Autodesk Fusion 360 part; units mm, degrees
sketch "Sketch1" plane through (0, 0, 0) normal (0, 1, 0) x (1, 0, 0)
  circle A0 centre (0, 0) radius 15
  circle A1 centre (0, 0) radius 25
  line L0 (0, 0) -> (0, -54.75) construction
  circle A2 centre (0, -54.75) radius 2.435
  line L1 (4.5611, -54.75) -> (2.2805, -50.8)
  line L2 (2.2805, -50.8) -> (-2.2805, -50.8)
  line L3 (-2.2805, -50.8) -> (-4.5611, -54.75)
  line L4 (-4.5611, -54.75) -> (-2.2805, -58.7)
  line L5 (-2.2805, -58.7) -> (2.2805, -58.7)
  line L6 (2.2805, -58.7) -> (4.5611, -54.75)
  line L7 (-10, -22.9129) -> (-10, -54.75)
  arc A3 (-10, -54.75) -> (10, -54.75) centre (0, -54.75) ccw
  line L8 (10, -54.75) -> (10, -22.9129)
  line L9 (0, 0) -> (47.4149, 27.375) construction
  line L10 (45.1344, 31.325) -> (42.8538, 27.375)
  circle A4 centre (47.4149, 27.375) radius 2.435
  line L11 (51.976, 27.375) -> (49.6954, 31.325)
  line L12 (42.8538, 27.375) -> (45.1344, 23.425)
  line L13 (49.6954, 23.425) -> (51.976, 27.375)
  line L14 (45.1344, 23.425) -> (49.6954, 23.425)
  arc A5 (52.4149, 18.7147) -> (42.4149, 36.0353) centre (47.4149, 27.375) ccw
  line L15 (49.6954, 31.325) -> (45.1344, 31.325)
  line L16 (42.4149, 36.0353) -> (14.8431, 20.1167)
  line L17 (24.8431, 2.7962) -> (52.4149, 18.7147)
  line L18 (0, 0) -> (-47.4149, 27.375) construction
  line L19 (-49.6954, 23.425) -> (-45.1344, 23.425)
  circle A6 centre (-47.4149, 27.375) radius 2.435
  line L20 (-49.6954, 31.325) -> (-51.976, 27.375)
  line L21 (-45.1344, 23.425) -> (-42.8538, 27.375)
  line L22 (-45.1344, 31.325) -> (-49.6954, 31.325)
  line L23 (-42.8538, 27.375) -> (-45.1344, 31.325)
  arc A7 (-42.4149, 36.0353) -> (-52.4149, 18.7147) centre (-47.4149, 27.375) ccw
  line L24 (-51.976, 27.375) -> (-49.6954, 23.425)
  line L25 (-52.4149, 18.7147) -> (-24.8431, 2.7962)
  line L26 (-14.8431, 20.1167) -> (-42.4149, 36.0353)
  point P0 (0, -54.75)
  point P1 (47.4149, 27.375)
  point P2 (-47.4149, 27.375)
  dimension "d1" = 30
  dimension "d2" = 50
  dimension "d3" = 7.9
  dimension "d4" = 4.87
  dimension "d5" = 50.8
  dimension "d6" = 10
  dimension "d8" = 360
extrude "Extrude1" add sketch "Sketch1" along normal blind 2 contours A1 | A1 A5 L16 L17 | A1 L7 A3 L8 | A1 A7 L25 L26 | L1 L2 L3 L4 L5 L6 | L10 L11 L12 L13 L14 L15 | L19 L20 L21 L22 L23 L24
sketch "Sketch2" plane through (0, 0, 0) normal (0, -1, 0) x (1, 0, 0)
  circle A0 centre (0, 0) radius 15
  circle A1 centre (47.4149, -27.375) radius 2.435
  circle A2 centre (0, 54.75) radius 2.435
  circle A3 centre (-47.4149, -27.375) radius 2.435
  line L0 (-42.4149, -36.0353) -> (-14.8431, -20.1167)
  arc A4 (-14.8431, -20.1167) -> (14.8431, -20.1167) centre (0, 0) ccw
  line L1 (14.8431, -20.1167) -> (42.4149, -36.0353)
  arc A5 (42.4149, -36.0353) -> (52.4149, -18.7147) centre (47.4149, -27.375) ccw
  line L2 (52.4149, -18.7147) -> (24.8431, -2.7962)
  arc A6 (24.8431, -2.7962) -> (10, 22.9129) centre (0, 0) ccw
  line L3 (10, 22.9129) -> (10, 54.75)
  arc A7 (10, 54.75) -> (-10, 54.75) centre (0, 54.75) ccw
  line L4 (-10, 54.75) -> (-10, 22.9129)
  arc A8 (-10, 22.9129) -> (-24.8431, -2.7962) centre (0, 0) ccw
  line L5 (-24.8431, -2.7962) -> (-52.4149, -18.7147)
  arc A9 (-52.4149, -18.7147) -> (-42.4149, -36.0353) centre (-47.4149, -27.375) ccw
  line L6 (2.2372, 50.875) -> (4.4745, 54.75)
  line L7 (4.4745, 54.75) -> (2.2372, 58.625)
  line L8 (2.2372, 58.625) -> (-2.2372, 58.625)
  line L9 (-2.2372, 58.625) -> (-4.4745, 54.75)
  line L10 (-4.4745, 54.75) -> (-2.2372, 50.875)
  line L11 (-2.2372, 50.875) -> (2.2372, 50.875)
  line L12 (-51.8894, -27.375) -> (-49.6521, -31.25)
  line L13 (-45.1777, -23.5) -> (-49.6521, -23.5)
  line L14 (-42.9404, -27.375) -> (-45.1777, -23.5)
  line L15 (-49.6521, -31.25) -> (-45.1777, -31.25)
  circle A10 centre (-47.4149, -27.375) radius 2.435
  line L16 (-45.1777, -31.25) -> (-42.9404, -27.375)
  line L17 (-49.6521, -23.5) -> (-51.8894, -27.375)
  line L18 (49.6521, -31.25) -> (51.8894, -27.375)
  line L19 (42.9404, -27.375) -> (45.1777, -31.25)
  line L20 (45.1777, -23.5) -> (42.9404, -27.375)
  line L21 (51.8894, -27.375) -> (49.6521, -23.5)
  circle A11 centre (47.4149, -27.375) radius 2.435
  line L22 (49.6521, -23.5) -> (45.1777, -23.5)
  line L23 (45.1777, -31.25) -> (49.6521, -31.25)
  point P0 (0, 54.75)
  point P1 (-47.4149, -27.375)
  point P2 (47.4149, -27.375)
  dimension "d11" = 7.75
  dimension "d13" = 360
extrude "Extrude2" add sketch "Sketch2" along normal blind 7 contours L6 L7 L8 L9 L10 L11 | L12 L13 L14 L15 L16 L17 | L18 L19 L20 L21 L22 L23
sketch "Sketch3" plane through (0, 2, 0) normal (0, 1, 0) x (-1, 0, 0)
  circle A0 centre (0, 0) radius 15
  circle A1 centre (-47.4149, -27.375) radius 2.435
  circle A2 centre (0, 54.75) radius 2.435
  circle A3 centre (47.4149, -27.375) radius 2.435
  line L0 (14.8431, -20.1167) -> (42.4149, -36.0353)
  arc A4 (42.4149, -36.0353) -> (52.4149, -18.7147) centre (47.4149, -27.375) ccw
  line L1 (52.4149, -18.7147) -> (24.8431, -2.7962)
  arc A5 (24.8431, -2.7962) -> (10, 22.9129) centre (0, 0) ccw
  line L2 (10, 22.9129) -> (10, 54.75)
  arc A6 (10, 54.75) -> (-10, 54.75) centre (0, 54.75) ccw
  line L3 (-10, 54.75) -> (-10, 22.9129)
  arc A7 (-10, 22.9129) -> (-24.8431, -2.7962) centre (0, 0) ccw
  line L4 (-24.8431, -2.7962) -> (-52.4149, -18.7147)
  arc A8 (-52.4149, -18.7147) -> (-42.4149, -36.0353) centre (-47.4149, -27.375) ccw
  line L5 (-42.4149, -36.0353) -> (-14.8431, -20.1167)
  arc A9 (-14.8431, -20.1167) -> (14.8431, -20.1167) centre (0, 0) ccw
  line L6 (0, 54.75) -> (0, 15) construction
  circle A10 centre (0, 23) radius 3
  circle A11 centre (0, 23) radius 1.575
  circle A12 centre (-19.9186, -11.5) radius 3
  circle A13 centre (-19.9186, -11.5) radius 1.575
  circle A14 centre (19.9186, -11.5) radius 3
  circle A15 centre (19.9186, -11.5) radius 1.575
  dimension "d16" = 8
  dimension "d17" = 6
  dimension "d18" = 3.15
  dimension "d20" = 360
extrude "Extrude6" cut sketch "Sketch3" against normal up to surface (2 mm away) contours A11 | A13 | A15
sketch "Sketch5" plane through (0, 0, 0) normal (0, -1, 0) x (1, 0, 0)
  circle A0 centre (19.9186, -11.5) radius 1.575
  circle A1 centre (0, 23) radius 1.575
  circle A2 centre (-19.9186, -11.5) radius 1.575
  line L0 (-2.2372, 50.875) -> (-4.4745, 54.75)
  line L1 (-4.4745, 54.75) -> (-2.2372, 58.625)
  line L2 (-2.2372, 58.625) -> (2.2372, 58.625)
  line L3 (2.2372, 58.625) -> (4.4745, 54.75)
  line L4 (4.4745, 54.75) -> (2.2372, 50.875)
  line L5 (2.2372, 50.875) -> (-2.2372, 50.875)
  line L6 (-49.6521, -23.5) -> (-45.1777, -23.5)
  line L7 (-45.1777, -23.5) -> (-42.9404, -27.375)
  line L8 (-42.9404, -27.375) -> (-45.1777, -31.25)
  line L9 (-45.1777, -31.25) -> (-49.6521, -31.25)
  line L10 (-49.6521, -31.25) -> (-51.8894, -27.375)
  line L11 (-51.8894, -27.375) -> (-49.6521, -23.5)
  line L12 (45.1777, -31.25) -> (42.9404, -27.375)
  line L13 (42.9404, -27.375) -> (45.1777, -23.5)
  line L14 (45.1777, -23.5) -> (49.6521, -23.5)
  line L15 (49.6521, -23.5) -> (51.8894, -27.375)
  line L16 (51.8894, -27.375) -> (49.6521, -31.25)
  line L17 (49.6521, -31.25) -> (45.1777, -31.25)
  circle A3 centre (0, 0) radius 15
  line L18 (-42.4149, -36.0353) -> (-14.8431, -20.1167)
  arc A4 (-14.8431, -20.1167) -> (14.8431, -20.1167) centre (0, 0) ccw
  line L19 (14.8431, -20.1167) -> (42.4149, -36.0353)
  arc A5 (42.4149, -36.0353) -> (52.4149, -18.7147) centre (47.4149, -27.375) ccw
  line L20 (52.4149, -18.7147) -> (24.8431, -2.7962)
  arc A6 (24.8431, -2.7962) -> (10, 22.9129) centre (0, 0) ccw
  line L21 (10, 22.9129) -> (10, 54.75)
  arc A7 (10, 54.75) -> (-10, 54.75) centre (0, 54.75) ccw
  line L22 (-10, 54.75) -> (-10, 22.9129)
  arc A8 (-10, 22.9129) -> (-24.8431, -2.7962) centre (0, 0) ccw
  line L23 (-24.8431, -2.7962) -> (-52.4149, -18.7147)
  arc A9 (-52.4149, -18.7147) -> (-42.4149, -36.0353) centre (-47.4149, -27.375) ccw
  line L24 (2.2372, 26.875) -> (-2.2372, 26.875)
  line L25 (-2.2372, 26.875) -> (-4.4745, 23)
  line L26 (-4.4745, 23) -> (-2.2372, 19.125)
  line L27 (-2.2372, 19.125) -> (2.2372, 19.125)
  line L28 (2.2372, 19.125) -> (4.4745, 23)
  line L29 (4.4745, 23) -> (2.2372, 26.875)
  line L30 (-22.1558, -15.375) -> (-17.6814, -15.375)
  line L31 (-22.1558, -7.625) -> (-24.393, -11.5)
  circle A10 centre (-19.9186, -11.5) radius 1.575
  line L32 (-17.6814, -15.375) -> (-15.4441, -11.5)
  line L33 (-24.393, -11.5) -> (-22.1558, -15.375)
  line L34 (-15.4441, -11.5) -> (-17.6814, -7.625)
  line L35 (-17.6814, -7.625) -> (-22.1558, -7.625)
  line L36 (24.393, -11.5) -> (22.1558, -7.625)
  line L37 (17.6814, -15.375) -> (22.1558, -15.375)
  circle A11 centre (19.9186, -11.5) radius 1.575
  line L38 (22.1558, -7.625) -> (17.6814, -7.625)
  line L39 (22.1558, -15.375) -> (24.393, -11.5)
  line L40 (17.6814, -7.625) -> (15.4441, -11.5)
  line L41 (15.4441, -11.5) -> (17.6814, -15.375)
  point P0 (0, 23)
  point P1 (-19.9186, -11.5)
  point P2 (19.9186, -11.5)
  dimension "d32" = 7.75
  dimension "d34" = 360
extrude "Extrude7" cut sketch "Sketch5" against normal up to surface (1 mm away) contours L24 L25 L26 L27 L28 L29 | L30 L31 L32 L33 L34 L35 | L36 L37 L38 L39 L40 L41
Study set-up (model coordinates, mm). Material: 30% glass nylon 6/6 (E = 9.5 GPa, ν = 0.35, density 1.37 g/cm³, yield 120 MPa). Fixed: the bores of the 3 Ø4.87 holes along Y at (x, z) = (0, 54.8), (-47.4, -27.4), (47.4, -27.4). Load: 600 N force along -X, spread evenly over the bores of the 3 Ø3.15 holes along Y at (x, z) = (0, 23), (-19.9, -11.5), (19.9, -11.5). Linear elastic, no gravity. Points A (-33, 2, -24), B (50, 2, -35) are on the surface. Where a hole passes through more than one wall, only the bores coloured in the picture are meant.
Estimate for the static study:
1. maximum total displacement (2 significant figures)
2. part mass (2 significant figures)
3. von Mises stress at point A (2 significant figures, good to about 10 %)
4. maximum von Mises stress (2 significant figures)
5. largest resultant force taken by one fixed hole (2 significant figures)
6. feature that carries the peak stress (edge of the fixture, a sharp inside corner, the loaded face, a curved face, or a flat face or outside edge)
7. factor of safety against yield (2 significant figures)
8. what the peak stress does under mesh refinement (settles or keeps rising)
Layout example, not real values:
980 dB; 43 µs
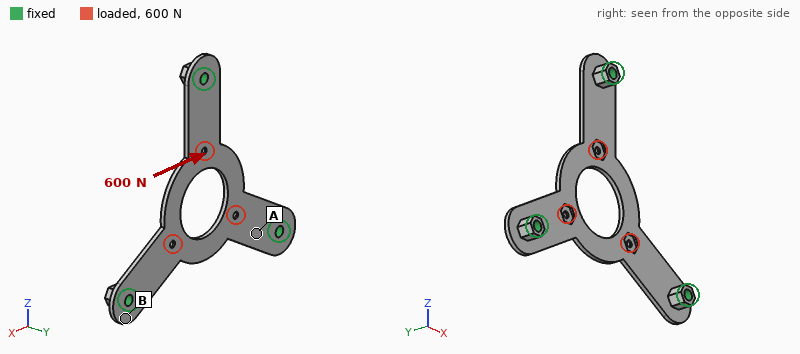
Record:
0.16 mm; 10 g; 7.9 MPa; 38 MPa; 300 N; the loaded face; 3.1; settles
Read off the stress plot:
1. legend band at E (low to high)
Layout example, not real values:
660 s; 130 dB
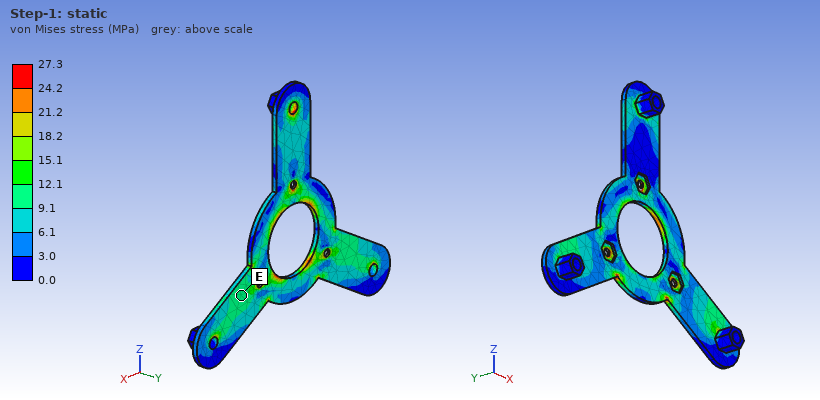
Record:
9.1 to 12.1 MPa
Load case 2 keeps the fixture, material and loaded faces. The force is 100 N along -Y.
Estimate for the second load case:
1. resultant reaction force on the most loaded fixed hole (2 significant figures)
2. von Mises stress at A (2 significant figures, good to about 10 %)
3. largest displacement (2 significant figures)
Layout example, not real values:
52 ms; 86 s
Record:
39 N; 21 MPa; 1.7 mm
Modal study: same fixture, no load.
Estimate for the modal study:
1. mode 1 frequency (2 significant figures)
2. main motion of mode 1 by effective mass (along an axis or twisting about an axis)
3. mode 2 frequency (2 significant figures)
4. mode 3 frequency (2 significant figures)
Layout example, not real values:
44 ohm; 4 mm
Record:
600 Hz; along Y; 1100 Hz; 1100 Hz
